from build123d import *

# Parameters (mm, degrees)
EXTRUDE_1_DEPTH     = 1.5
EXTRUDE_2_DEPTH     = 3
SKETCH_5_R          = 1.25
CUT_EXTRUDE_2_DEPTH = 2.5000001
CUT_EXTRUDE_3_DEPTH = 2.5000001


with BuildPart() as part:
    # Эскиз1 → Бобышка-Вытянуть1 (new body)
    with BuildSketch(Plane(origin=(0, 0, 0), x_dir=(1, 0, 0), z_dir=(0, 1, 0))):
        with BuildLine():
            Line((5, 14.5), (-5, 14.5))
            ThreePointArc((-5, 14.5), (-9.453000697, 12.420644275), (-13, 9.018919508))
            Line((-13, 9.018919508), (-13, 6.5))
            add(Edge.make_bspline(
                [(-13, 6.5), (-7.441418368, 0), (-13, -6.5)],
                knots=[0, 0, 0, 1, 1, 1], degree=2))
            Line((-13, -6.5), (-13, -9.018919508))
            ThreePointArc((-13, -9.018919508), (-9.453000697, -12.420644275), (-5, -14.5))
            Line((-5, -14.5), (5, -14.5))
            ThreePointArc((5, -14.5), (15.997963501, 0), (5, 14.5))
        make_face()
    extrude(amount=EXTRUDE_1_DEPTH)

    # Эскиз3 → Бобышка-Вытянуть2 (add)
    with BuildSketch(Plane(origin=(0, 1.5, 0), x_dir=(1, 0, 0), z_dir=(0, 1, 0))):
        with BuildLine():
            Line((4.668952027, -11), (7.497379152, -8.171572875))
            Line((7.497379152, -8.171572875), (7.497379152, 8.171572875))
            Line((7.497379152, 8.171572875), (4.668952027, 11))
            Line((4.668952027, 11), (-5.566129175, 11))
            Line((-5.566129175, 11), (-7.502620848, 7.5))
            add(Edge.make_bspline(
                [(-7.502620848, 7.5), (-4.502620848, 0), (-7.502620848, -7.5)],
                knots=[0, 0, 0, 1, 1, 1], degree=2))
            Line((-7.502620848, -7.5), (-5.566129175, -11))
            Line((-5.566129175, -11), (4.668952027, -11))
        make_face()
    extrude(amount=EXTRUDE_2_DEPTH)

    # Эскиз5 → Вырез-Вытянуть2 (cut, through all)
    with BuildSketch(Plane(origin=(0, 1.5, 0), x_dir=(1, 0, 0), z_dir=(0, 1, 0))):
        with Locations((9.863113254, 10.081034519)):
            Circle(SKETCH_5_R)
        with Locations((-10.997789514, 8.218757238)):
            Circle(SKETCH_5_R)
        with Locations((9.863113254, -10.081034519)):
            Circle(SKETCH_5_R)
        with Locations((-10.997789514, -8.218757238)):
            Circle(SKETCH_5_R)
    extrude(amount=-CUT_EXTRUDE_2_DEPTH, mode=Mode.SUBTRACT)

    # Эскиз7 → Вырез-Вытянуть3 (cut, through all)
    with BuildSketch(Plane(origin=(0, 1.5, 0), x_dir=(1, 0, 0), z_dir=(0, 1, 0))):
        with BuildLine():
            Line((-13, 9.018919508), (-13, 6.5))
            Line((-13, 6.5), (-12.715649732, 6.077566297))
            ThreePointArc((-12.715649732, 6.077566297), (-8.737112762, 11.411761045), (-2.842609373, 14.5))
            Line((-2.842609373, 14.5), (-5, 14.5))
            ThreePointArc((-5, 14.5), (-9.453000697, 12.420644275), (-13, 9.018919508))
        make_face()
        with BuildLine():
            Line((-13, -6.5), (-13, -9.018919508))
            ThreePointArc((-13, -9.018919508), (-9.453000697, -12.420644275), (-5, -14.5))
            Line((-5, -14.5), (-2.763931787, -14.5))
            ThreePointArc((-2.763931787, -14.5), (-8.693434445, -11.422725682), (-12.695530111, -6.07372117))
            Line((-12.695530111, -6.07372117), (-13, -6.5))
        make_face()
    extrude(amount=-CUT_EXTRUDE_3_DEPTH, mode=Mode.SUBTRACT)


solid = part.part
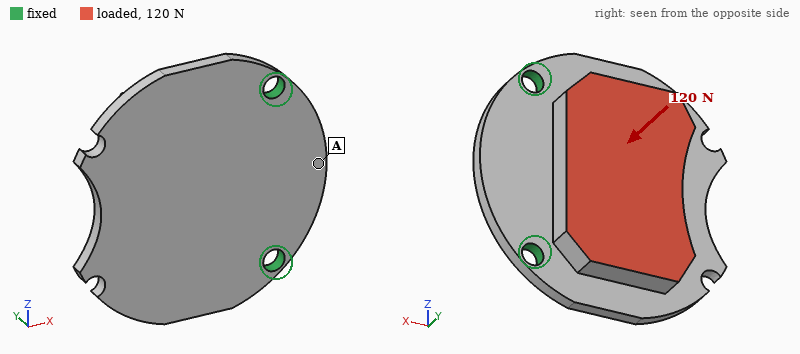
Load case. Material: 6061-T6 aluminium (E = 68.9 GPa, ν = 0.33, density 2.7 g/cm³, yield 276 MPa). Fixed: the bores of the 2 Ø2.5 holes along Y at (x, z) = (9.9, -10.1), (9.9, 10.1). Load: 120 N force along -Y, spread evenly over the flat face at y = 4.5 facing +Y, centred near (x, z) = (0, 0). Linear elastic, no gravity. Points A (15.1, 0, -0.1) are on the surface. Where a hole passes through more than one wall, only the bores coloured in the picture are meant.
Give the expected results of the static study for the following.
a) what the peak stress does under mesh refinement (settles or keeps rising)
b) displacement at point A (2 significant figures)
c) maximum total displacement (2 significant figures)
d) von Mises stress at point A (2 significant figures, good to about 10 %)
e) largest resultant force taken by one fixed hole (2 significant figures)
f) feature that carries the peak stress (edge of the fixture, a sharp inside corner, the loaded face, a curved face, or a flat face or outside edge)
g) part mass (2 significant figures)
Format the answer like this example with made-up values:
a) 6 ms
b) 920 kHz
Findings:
a) keeps rising
b) 0.022 mm
c) 0.15 mm
d) 21 MPa
e) 66 N
f) edge of the fixture
g) 5.1 g
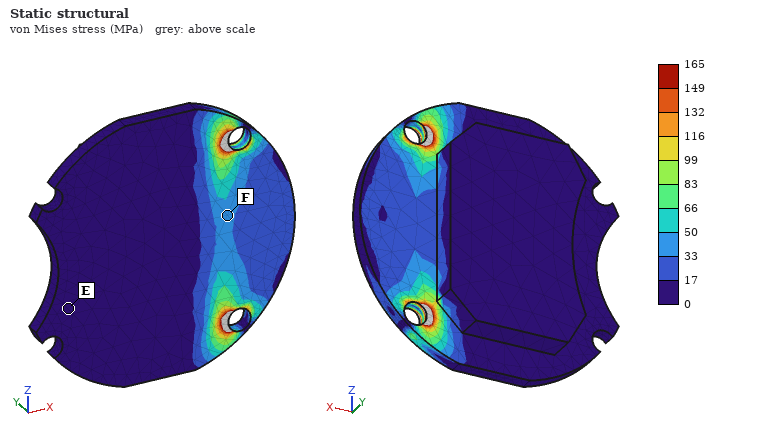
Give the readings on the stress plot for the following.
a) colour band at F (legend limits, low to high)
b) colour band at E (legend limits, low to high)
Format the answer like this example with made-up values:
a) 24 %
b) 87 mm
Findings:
a) 33 to 50 MPa
b) 0 to 17 MPa
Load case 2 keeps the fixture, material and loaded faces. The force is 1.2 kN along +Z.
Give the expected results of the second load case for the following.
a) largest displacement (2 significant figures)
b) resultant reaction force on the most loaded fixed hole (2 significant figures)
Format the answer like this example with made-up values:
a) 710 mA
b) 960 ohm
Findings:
a) 28 µm
b) 840 N
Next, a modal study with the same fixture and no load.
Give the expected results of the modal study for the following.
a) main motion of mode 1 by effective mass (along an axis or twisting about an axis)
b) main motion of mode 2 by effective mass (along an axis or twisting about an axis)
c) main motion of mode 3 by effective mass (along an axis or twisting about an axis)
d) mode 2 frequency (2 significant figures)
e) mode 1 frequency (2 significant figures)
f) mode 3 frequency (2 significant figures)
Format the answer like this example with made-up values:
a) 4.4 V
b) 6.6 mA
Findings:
a) along Y
b) twisting about X
c) along Y
d) 13 kHz
e) 2800 Hz
f) 21 kHz
